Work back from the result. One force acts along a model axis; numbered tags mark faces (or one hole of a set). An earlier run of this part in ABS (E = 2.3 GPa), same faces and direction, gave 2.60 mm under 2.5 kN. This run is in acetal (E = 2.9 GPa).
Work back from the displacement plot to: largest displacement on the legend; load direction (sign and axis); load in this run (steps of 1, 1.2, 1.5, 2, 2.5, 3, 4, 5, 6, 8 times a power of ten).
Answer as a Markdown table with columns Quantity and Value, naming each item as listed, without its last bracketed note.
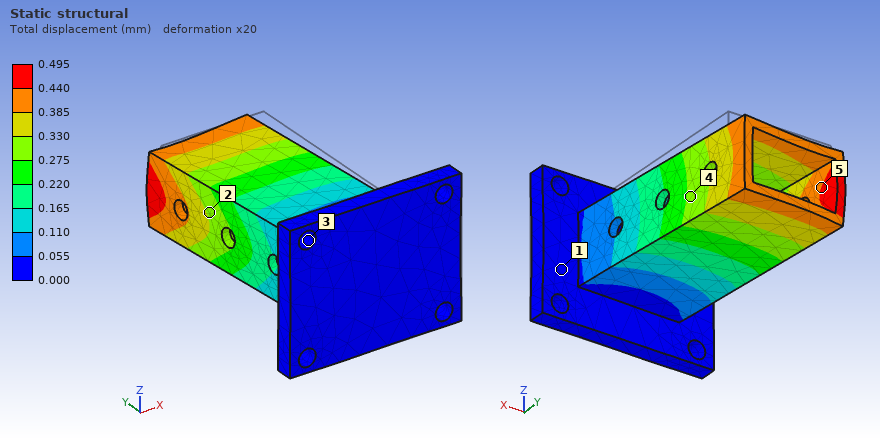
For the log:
| Quantity | Value |
|---|---|
| largest displacement on the legend | 0.495 mm |
| load direction | -X |
| load in this run | 600 N |
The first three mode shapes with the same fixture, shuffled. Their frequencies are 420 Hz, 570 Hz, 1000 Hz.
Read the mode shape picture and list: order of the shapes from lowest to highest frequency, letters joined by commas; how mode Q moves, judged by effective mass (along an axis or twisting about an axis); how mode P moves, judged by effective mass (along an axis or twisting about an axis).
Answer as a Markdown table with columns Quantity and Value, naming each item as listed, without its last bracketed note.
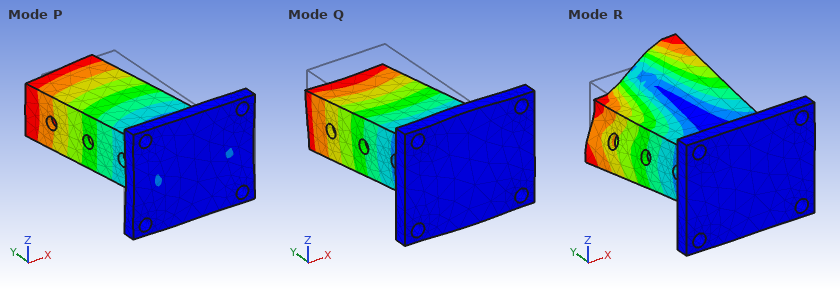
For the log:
| Quantity | Value |
|---|---|
| order of the shapes from lowest to highest frequency, letters joined by commas | Q, P, R |
| how mode Q moves, judged by effective mass | along Z |
| how mode P moves, judged by effective mass | along X |
